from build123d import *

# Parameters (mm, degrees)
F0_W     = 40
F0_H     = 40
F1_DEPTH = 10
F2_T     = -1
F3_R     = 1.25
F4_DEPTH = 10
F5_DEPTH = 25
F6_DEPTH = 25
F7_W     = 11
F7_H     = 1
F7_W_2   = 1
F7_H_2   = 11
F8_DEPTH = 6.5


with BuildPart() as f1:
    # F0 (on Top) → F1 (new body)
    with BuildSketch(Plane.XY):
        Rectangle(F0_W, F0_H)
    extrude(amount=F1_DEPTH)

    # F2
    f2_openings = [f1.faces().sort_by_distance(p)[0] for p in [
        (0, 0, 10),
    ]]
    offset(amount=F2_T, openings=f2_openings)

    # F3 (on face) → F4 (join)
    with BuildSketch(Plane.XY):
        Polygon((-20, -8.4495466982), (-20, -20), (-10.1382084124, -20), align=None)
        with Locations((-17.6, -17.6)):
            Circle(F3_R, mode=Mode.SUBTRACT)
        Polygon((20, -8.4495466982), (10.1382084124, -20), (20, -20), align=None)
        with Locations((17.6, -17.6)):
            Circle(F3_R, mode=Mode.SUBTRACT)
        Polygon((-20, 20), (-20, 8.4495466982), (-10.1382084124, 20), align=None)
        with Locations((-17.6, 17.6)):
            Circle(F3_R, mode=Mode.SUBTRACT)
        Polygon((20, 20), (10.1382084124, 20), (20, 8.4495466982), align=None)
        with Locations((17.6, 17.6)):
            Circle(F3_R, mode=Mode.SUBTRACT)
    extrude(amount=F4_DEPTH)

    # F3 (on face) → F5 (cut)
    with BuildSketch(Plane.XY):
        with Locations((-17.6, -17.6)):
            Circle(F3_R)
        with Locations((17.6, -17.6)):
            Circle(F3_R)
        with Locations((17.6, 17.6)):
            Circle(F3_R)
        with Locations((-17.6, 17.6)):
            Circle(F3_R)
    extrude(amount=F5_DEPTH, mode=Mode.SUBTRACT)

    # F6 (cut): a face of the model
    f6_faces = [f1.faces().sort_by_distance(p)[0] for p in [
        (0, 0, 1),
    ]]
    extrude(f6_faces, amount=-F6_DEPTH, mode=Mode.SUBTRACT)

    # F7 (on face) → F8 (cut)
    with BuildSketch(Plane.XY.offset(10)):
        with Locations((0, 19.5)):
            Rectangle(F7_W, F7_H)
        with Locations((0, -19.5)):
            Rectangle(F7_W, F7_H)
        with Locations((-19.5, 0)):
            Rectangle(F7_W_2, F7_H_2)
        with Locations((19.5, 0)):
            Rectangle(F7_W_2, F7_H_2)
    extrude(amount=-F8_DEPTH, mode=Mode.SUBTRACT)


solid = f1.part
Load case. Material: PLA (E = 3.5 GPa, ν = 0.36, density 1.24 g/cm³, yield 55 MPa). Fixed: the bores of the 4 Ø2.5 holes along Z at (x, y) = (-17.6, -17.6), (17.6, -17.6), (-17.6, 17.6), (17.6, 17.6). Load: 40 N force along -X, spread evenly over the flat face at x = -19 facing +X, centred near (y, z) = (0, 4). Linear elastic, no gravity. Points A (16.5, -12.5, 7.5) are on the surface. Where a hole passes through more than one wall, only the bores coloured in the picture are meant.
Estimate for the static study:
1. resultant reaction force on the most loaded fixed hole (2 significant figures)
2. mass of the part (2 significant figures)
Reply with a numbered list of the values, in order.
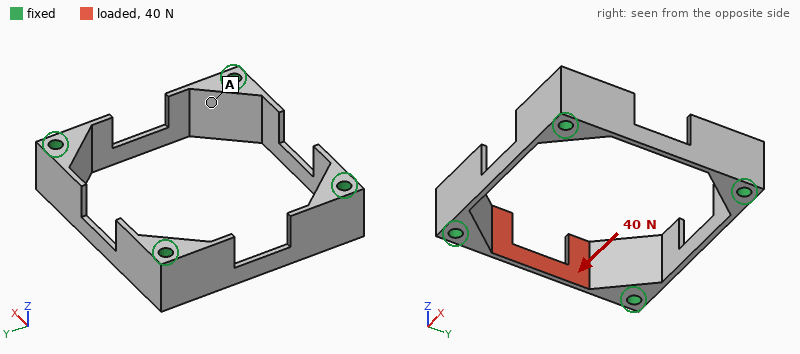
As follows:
1. 23 N
2. 3.2 g
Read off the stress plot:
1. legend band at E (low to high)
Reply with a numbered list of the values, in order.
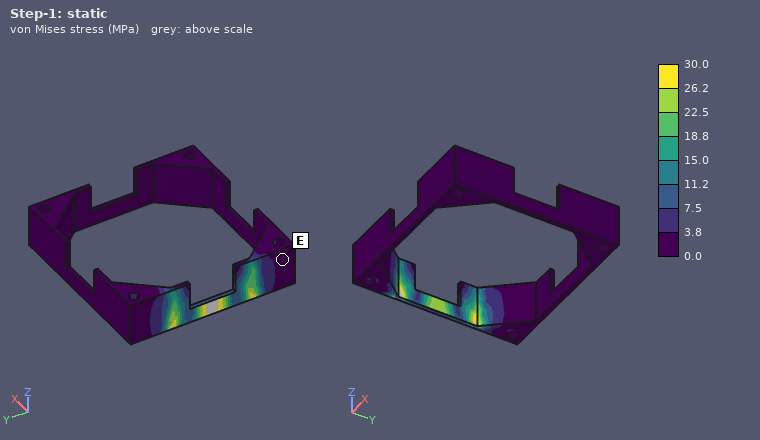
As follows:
1. 0.0 to 3.8 MPa
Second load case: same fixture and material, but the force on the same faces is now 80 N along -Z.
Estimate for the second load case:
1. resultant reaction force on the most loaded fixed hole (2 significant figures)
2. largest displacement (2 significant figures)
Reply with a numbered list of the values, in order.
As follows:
1. 42 N
2. 0.12 mm
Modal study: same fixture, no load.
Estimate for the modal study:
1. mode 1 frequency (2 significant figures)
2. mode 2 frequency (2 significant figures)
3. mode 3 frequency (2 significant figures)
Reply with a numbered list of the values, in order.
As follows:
1. 3800 Hz
2. 3900 Hz
3. 4600 Hz
